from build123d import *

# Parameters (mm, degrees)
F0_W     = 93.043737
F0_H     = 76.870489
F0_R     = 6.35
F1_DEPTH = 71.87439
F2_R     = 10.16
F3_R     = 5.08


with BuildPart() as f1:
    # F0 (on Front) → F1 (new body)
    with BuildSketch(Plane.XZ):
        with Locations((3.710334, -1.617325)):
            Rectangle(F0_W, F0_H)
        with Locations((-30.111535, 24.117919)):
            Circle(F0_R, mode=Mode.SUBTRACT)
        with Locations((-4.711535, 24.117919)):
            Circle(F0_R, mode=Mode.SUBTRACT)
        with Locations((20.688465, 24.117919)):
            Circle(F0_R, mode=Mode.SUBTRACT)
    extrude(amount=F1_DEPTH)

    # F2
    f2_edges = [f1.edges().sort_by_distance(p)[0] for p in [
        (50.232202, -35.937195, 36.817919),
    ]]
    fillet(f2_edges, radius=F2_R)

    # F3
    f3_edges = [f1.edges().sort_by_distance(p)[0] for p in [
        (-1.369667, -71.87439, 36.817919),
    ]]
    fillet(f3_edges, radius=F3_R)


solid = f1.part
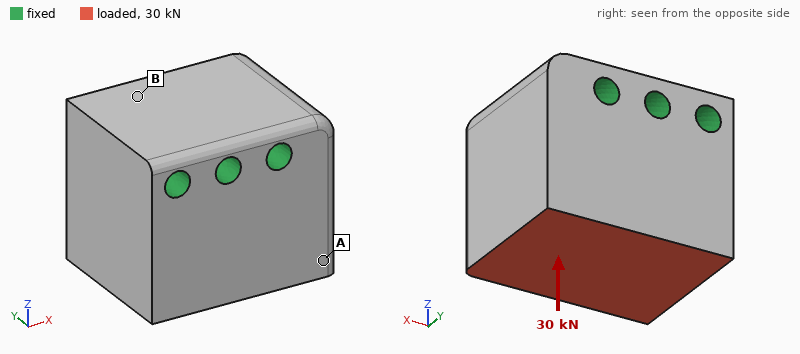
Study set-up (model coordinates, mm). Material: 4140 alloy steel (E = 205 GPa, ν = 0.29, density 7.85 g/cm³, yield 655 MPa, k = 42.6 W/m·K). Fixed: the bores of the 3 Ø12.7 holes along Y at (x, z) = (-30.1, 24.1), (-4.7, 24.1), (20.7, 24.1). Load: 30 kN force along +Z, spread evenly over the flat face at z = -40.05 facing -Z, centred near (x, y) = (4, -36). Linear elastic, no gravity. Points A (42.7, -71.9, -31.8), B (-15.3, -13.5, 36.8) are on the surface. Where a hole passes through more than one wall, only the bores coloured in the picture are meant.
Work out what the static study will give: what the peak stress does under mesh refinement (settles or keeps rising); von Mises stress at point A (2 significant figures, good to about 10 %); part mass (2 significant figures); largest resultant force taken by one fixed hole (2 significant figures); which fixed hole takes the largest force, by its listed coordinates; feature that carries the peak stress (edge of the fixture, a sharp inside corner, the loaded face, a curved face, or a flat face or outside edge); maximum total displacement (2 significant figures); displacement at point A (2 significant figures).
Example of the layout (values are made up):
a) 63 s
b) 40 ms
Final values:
a) keeps rising
b) 4.4 MPa
c) 3.8 kg
d) 15 kN
e) (20.7, 24.1)
f) edge of the fixture
g) 2.2 µm
h) 1.9 µm
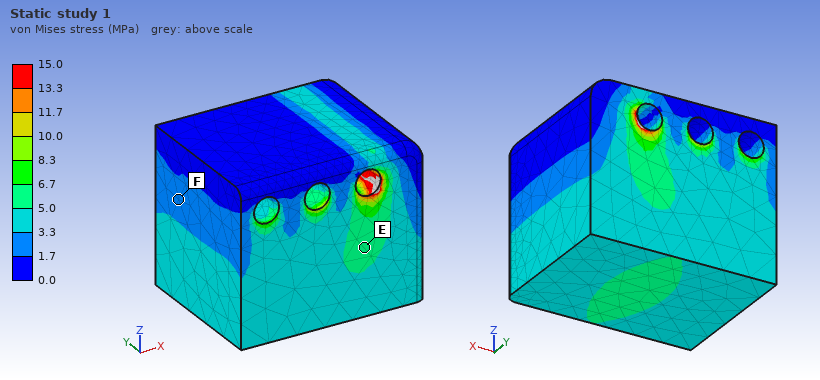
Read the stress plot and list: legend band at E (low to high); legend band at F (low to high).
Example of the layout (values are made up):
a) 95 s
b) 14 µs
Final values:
a) 5.0 to 6.7 MPa
b) 1.7 to 3.3 MPa
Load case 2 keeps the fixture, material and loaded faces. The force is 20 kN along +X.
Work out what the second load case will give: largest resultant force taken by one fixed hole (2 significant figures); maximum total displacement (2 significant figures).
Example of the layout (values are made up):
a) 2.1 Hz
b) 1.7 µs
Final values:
a) 22 kN
b) 7.2 µm
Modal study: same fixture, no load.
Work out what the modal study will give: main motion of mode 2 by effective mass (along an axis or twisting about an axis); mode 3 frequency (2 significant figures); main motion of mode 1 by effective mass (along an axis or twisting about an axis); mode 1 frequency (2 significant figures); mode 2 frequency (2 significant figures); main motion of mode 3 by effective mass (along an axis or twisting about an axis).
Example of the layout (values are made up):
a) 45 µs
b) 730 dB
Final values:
a) along Y
b) 12 kHz
c) along X
d) 8400 Hz
e) 8900 Hz
f) twisting about Z
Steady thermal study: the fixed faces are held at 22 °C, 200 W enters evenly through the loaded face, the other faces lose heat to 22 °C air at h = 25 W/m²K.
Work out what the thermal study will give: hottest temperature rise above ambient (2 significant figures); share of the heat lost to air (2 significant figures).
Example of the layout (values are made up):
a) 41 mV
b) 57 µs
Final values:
a) 43 K
b) 5.5 %
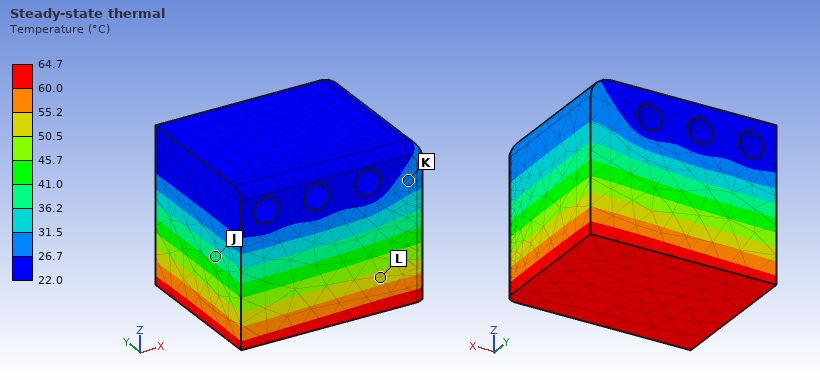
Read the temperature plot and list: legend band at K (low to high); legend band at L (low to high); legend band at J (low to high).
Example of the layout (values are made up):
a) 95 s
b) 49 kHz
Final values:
a) 26.7 to 31.5 °C
b) 50.5 to 55.2 °C
c) 36.2 to 41.0 °C
